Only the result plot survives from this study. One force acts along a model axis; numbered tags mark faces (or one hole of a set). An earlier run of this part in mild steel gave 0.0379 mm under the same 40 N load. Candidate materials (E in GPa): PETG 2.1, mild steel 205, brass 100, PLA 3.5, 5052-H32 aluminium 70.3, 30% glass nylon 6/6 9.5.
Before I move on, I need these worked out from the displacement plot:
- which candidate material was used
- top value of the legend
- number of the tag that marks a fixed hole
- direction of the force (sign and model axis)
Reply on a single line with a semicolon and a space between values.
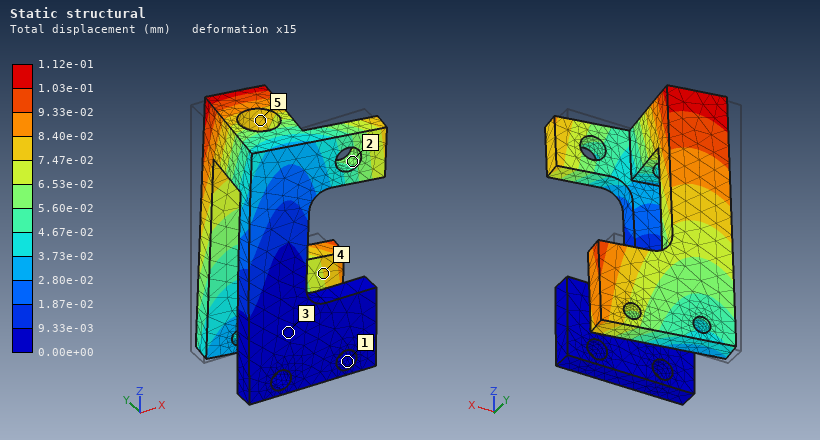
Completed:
5052-H32 aluminium; 1.12e-01 mm; 1; +X
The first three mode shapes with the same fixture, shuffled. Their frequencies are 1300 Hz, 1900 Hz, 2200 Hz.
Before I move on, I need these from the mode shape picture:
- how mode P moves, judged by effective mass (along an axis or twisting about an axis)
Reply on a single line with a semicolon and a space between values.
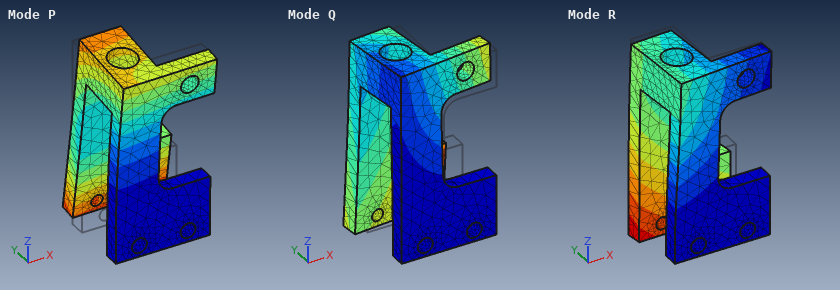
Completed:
along Z
